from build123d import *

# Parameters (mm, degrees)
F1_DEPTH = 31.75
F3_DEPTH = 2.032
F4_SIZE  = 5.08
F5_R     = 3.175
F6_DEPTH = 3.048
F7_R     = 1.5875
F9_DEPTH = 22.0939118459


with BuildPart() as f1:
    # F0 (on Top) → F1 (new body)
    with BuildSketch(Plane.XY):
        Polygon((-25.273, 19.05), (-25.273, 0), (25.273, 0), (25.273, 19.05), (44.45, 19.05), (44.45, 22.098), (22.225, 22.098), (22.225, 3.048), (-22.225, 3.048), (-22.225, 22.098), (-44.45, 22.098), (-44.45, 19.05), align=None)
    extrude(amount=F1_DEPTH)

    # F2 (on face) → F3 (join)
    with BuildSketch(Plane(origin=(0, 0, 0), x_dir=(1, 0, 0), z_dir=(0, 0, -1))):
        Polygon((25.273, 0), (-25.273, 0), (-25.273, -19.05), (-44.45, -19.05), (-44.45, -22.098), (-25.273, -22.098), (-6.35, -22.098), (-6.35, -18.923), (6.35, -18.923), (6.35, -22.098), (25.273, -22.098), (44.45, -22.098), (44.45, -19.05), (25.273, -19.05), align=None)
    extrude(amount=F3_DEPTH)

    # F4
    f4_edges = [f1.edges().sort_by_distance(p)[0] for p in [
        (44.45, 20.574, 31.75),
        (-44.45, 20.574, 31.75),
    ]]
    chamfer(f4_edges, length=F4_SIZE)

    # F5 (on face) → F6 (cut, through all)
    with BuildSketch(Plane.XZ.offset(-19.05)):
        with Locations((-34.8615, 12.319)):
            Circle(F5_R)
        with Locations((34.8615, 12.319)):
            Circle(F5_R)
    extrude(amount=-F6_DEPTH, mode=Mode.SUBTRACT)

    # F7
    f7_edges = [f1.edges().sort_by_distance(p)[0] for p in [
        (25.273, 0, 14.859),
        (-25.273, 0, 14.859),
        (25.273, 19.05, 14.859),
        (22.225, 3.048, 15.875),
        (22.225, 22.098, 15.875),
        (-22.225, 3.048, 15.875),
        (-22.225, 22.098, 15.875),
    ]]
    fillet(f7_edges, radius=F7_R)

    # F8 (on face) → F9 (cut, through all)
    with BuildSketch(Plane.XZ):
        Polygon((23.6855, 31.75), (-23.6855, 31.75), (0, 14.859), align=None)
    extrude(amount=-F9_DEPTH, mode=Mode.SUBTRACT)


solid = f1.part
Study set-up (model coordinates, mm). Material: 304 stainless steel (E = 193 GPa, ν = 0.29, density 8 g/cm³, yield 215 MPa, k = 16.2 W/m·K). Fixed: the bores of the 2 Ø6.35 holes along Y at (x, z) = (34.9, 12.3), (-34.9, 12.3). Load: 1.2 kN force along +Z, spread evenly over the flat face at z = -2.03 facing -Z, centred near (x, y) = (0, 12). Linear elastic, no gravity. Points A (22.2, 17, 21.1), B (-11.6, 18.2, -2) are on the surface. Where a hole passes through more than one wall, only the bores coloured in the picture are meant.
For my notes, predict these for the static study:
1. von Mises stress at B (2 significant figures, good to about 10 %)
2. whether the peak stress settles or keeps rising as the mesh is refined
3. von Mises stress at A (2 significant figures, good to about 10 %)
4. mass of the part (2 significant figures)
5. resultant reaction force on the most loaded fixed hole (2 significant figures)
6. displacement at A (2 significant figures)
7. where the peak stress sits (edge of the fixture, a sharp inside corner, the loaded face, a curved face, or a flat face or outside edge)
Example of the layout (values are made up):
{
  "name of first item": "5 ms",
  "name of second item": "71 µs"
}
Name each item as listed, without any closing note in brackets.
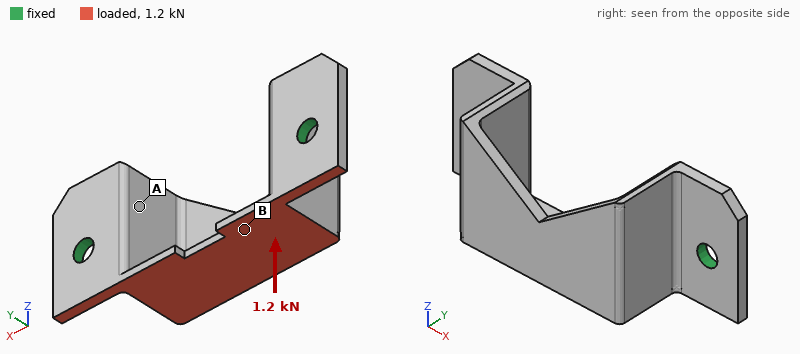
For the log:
{
  "von Mises stress at B": "56 MPa",
  "whether the peak stress settles or keeps rising as the mesh is refined": "keeps rising",
  "von Mises stress at A": "22 MPa",
  "mass of the part": "110 g",
  "resultant reaction force on the most loaded fixed hole": "640 N",
  "displacement at A": "16 µm",
  "where the peak stress sits": "edge of the fixture"
}
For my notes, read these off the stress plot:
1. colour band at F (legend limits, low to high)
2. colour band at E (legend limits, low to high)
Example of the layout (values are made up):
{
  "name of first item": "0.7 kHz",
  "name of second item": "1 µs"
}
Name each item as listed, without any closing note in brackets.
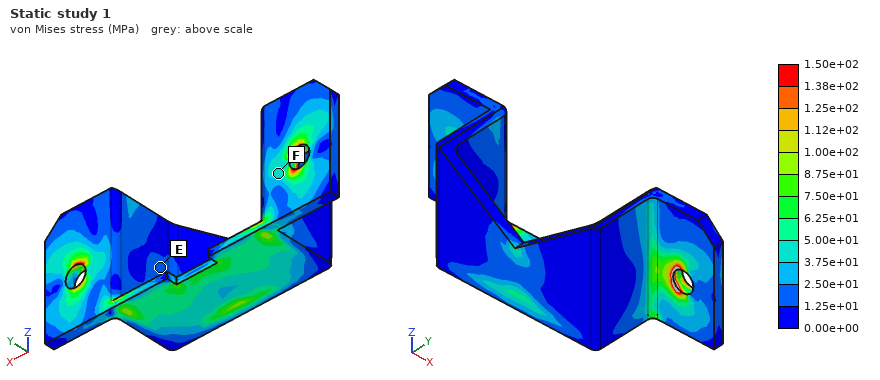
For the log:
{
  "colour band at F": "3.75e+01 to 5.00e+01 MPa",
  "colour band at E": "1.25e+01 to 2.50e+01 MPa"
}
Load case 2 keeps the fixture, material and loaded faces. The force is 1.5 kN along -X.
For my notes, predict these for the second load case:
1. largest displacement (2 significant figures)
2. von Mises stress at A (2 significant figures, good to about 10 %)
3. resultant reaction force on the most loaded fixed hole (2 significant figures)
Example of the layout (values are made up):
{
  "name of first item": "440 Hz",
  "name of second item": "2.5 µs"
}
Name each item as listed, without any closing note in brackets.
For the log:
{
  "largest displacement": "13 µm",
  "von Mises stress at A": "16 MPa",
  "resultant reaction force on the most loaded fixed hole": "800 N"
}
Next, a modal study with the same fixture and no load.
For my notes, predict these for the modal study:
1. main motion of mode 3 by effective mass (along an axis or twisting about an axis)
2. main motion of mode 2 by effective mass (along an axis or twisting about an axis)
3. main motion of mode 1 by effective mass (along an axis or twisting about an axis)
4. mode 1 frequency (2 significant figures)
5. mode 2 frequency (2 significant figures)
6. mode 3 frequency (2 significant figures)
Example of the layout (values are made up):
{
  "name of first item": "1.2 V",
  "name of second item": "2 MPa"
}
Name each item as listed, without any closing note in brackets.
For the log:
{
  "main motion of mode 3 by effective mass": "along Y",
  "main motion of mode 2 by effective mass": "along X",
  "main motion of mode 1 by effective mass": "along Z",
  "mode 1 frequency": "2600 Hz",
  "mode 2 frequency": "3500 Hz",
  "mode 3 frequency": "6300 Hz"
}
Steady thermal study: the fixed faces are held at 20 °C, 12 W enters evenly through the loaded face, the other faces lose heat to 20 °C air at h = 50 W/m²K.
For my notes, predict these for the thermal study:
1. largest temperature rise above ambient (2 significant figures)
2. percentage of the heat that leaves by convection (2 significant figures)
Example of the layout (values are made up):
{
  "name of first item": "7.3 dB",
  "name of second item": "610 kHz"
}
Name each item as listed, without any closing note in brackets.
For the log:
{
  "largest temperature rise above ambient": "61 K",
  "percentage of the heat that leaves by convection": "70 %"
}
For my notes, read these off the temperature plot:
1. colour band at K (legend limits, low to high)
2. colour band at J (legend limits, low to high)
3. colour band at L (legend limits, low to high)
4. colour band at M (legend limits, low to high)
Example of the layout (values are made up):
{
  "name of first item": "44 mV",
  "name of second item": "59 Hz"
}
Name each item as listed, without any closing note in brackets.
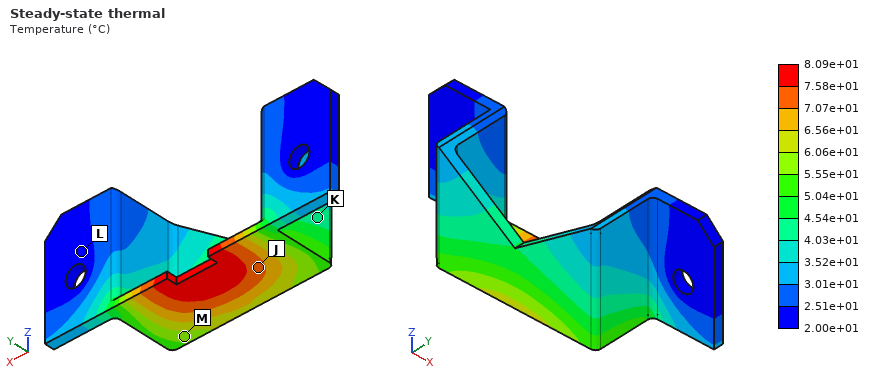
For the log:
{
  "colour band at K": "4.03e+01 to 4.54e+01 °C",
  "colour band at J": "7.07e+01 to 7.58e+01 °C",
  "colour band at L": "2.00e+01 to 2.51e+01 °C",
  "colour band at M": "5.55e+01 to 6.06e+01 °C"
}
